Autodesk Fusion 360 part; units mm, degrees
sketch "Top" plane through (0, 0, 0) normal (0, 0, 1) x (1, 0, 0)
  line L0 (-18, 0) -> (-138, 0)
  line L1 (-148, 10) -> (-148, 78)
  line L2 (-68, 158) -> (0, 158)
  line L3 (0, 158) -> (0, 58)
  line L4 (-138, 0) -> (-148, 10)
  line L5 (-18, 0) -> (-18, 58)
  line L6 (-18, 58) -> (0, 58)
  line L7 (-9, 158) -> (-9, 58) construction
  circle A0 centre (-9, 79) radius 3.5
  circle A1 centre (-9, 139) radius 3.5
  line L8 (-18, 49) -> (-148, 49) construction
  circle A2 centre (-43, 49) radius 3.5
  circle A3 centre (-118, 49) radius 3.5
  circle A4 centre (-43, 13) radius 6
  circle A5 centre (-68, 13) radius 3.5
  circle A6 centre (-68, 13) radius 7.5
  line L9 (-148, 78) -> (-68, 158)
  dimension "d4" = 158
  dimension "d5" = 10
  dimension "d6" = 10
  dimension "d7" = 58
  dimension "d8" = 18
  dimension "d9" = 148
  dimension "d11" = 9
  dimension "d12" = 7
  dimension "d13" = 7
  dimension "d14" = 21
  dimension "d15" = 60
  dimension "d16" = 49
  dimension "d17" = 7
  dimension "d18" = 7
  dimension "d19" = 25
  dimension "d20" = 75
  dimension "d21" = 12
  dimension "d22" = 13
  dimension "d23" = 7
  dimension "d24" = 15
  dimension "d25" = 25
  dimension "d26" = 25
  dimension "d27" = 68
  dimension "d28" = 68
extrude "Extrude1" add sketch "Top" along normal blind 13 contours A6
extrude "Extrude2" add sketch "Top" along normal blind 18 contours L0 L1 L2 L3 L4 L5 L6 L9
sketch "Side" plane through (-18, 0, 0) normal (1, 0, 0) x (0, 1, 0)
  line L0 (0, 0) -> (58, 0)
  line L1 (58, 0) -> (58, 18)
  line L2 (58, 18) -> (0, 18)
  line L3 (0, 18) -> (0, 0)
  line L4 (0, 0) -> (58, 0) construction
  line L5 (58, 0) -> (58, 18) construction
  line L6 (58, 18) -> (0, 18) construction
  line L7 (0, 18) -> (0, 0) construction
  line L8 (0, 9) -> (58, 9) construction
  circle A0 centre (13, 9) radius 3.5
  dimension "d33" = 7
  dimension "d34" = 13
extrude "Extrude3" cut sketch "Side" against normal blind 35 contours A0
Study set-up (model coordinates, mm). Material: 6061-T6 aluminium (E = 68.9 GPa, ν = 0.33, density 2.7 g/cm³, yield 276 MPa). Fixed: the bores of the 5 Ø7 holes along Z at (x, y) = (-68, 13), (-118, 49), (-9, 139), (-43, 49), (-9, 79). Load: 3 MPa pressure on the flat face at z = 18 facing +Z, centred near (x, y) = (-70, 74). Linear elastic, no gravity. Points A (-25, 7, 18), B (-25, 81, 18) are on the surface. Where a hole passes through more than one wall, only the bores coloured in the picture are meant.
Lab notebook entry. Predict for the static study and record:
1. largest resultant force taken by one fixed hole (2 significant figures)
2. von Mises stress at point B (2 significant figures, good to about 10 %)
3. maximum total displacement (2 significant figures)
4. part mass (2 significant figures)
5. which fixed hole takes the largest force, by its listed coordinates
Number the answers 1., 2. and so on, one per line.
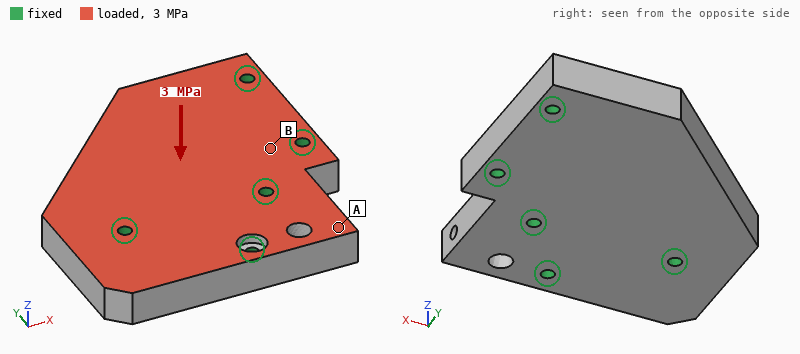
1. 21 kN
2. 38 MPa
3. 0.27 mm
4. 910 g
5. (-118, 49)
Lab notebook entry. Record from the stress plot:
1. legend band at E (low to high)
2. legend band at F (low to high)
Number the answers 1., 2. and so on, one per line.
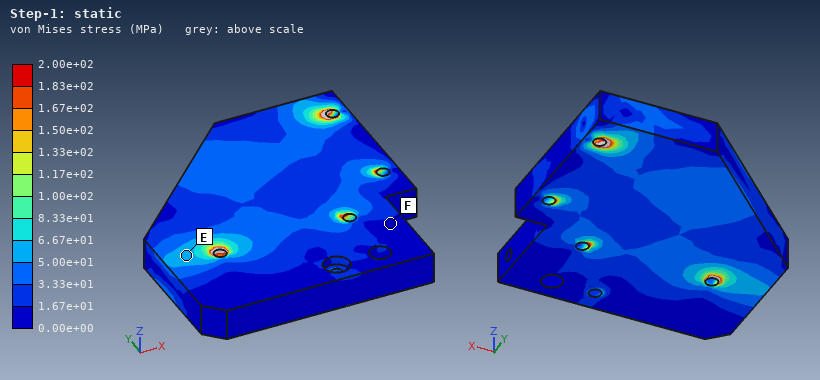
1. 5.00e+01 to 6.67e+01 MPa
2. 0.00e+00 to 1.67e+01 MPa
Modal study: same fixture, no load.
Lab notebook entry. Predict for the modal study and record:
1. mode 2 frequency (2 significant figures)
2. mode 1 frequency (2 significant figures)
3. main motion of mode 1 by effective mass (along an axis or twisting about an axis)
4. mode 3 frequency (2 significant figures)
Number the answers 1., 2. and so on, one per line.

1. 6000 Hz
2. 3100 Hz
3. along Z
4. 7200 Hz
